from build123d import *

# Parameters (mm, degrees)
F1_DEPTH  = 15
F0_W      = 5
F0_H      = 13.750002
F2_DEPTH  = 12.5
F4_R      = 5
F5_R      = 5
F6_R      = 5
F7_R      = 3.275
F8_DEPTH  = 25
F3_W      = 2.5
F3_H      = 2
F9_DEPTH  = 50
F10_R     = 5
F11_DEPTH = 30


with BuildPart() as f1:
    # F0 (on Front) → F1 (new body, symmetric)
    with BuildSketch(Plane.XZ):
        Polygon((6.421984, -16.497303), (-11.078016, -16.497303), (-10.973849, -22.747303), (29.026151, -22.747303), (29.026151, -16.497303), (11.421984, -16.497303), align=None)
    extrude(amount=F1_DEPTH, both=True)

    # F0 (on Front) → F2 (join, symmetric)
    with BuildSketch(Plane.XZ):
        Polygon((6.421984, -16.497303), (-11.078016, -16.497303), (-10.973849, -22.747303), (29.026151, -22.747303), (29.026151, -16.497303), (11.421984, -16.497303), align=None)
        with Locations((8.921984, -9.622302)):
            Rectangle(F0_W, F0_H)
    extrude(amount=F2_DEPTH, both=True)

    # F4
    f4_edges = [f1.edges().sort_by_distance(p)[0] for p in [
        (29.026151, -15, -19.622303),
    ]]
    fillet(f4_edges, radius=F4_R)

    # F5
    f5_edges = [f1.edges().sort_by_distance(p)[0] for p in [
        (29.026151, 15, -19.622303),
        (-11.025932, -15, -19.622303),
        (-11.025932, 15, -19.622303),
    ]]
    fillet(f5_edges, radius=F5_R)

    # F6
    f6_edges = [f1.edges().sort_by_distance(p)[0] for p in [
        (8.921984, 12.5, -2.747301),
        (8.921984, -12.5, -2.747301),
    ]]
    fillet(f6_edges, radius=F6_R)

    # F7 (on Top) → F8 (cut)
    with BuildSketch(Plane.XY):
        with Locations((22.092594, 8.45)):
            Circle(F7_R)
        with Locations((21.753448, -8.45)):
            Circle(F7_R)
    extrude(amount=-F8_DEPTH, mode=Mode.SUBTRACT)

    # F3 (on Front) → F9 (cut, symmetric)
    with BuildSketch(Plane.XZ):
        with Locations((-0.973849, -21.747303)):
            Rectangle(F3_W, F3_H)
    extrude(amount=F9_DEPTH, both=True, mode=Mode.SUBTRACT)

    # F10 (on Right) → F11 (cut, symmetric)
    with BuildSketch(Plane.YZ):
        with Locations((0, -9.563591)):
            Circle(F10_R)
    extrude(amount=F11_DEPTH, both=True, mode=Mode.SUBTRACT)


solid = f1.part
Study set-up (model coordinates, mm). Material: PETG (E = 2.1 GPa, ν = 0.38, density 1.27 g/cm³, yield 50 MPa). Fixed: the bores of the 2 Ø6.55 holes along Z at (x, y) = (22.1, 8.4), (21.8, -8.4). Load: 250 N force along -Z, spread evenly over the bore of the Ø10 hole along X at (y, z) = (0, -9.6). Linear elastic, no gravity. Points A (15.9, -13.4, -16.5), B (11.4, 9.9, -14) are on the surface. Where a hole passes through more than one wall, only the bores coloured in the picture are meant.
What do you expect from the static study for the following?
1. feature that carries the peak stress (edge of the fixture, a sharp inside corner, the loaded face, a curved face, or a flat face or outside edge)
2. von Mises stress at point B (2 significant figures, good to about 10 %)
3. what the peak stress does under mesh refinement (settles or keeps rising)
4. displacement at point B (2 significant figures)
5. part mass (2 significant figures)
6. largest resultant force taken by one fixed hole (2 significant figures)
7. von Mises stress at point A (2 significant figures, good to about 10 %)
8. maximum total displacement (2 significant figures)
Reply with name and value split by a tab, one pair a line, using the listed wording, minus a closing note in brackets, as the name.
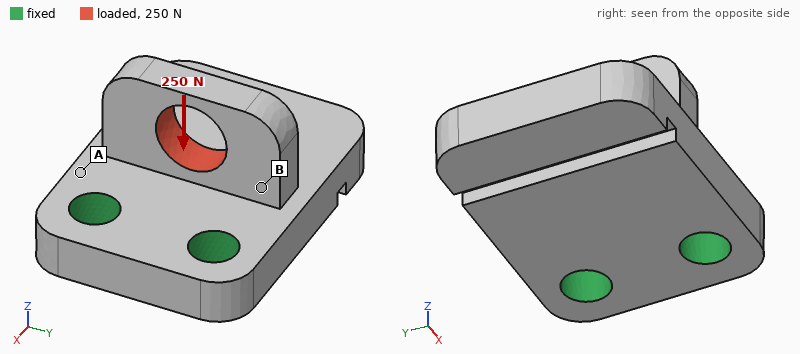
feature that carries the peak stress	edge of the fixture
von Mises stress at point B	2.9 MPa
what the peak stress does under mesh refinement	keeps rising
displacement at point B	0.11 mm
part mass	10 g
largest resultant force taken by one fixed hole	130 N
von Mises stress at point A	7.5 MPa
maximum total displacement	0.35 mm
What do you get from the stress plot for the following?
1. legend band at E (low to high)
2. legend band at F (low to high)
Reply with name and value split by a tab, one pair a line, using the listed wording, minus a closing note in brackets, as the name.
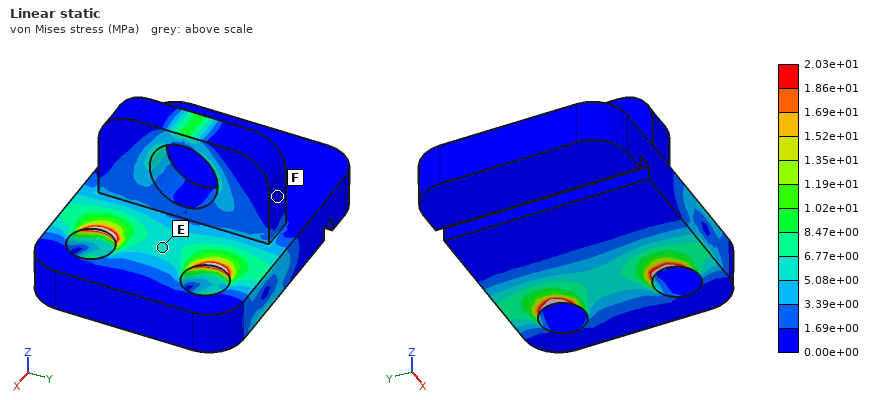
legend band at E	5.08e+00 to 6.77e+00 MPa
legend band at F	0.00e+00 to 1.69e+00 MPa
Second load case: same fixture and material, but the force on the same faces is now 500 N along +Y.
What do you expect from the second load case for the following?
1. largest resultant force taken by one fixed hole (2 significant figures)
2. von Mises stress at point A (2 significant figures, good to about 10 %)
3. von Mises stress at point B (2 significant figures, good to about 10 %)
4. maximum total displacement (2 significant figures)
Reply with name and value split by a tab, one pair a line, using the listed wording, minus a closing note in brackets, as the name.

largest resultant force taken by one fixed hole	440 N
von Mises stress at point A	10 MPa
von Mises stress at point B	12 MPa
maximum total displacement	0.43 mm
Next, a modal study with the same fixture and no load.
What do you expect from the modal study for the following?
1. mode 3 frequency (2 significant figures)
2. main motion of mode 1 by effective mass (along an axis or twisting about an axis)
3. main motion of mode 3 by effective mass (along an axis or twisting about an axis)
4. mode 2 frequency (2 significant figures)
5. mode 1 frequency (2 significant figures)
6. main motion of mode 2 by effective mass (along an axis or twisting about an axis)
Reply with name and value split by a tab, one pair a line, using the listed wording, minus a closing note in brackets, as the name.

mode 3 frequency	3900 Hz
main motion of mode 1 by effective mass	along Z
main motion of mode 3 by effective mass	along Y
mode 2 frequency	2900 Hz
mode 1 frequency	1300 Hz
main motion of mode 2 by effective mass	twisting about X
